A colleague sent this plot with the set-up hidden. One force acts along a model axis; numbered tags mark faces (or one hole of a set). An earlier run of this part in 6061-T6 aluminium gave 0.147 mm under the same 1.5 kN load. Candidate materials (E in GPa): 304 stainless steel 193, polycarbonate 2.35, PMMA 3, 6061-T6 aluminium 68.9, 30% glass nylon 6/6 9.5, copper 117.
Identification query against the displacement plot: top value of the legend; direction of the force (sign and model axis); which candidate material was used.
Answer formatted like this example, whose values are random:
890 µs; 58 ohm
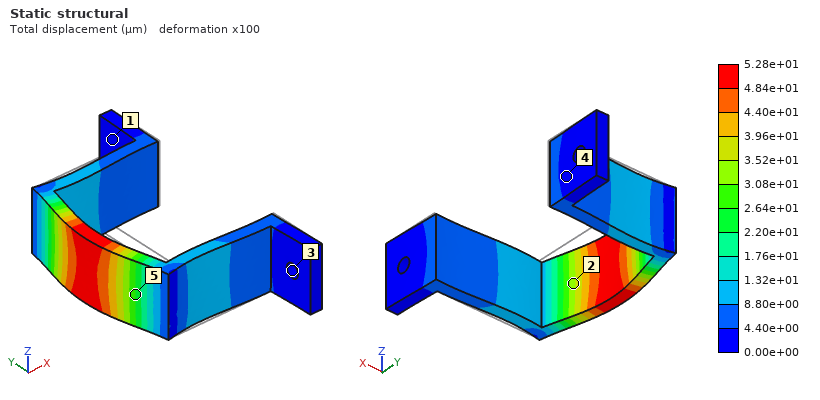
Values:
5.28e+01 µm; -X; 304 stainless steel
